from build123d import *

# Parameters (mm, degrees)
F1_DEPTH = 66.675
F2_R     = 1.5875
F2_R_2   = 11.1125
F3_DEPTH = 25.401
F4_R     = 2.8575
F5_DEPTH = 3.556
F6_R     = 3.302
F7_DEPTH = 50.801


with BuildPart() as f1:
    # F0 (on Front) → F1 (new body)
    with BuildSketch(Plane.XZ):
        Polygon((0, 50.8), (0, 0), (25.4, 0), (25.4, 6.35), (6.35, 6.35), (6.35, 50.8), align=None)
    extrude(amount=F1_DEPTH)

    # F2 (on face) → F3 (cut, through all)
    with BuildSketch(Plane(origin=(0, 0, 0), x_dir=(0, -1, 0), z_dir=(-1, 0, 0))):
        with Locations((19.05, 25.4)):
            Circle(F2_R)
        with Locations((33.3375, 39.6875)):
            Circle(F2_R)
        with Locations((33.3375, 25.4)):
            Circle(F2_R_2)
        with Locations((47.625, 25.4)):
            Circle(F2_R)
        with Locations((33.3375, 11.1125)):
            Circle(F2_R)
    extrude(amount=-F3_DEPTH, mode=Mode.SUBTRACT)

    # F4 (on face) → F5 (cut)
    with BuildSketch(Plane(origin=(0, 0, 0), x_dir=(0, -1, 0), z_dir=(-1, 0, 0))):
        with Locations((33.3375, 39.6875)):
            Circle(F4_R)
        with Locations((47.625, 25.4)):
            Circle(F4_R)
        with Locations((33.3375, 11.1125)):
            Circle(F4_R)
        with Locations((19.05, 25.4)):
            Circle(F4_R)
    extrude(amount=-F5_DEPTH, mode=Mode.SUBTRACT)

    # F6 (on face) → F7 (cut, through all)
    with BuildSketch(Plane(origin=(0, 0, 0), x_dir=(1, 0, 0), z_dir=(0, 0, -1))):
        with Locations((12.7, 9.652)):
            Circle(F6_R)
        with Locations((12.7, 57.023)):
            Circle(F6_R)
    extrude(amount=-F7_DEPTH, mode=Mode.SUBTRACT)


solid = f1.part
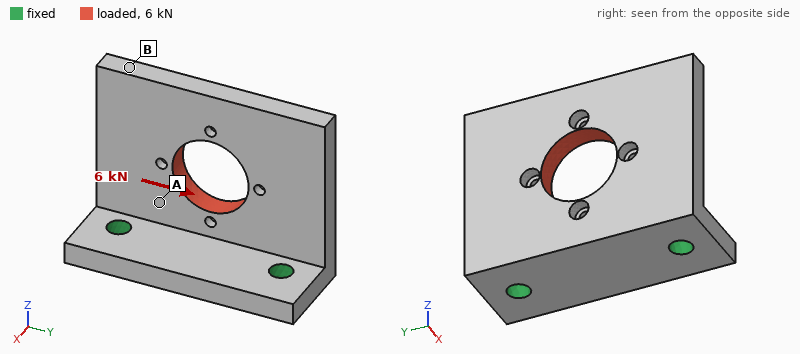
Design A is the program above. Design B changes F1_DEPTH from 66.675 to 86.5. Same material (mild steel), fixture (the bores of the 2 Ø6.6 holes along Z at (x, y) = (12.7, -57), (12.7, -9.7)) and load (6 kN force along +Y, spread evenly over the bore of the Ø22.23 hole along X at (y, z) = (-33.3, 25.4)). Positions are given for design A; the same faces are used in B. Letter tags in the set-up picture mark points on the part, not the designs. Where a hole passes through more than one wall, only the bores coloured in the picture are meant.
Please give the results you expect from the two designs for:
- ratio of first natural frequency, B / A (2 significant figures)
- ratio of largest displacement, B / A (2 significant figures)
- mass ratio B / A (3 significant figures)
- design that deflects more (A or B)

0.97
1.2
1.34
B
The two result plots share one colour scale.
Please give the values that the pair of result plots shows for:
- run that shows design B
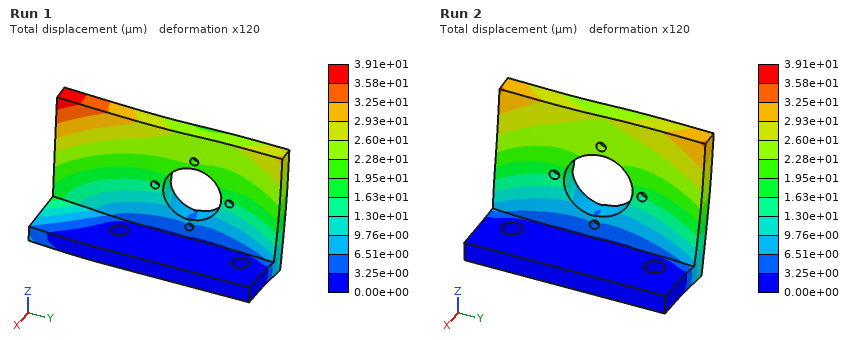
Run 1
